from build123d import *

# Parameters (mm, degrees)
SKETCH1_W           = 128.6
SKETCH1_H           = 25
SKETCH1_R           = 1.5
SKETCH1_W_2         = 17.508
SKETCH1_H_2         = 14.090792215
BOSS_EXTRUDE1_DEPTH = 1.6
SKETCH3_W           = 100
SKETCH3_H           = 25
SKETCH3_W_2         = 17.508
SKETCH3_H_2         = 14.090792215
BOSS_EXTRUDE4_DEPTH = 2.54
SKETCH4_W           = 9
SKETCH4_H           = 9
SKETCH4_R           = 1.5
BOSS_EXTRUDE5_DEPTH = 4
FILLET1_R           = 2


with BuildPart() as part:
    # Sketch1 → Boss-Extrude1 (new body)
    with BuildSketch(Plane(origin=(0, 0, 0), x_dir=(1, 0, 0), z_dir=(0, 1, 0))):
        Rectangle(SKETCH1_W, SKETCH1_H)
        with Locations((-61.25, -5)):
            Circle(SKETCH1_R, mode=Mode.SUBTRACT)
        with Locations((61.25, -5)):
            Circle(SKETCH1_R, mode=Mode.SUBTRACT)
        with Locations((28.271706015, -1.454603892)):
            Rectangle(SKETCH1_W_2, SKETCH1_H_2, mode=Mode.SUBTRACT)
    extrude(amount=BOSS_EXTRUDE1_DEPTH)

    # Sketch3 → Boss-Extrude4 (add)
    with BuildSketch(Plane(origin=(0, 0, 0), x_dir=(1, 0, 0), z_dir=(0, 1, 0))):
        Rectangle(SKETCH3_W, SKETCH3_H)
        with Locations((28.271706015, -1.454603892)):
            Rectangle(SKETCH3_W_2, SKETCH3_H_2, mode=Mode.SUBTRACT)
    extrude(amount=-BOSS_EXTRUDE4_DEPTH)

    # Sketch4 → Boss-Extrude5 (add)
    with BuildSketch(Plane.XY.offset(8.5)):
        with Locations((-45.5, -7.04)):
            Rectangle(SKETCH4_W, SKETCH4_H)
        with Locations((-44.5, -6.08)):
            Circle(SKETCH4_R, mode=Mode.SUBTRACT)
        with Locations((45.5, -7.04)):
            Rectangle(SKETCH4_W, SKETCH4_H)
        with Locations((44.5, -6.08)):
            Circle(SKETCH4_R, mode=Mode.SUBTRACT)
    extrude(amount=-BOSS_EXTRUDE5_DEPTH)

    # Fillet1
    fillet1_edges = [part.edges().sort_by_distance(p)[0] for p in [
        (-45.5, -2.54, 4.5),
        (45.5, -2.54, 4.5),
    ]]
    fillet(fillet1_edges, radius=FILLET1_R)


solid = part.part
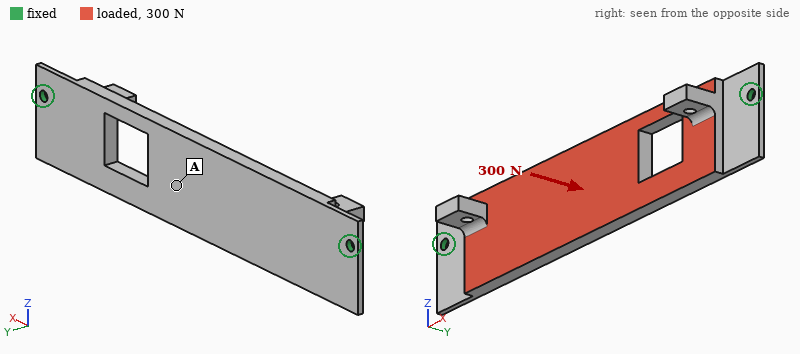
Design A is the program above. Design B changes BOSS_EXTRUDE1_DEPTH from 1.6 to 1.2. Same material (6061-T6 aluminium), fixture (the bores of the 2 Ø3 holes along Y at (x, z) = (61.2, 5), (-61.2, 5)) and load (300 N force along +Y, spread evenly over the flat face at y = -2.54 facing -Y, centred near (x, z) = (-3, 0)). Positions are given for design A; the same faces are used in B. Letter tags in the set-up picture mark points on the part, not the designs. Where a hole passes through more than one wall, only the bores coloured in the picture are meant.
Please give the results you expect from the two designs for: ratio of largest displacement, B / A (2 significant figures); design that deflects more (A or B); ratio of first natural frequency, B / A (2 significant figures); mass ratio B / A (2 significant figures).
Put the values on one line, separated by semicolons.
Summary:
1.6; B; 0.83; 0.89
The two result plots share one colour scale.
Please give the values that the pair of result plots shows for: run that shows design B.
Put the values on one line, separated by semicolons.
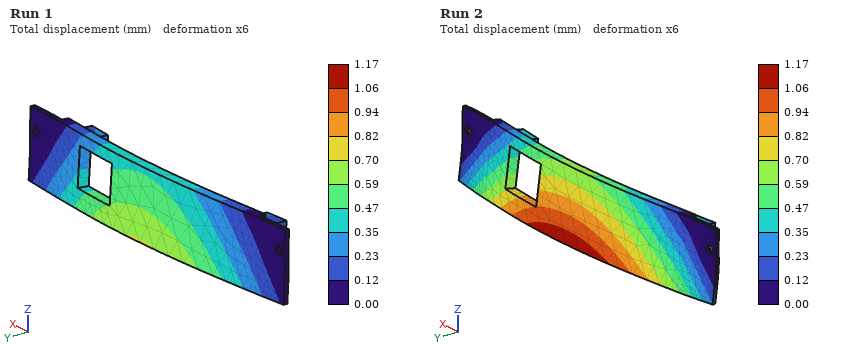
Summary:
Run 2
